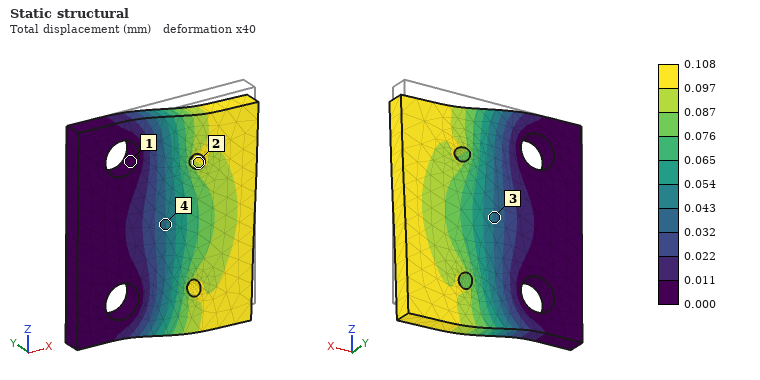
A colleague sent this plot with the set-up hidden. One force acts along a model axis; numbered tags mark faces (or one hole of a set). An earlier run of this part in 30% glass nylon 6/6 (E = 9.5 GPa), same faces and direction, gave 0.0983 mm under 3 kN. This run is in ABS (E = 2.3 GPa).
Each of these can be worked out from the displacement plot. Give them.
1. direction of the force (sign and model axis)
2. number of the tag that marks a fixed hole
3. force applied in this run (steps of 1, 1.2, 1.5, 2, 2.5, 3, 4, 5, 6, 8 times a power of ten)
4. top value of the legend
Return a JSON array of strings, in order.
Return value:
["-Z", "1", "800 N", "0.108 mm"]
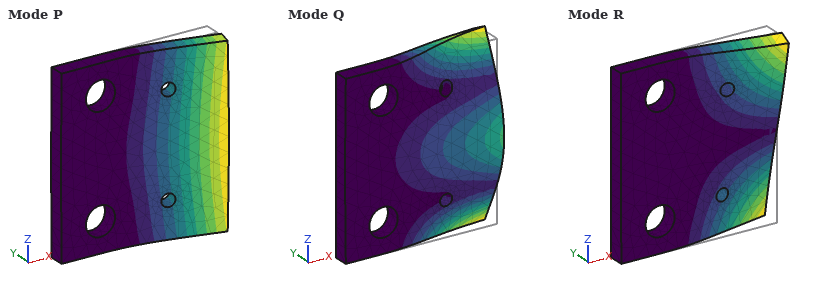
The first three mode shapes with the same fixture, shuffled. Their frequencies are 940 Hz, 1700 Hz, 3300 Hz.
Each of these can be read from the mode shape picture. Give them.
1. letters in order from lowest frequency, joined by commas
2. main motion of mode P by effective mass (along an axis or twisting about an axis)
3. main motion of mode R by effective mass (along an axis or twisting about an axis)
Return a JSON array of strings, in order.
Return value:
["P, R, Q", "along Y", "twisting about X"]
